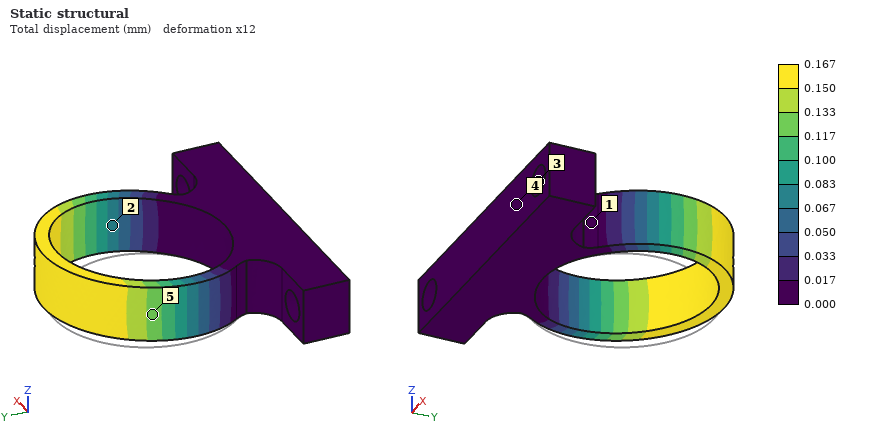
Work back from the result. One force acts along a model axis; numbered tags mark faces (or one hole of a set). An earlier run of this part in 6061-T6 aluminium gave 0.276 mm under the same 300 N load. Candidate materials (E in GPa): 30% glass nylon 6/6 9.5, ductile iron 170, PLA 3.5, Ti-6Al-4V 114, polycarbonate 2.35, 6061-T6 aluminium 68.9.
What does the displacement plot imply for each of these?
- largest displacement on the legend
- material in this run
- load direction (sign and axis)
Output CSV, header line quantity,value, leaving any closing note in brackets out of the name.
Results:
quantity,value
largest displacement on the legend,0.167 mm
material in this run,Ti-6Al-4V
load direction,+X
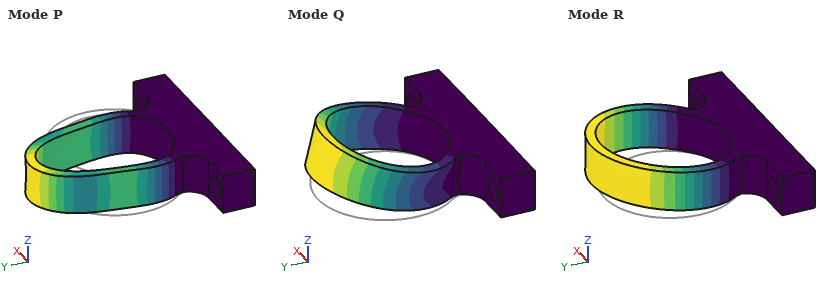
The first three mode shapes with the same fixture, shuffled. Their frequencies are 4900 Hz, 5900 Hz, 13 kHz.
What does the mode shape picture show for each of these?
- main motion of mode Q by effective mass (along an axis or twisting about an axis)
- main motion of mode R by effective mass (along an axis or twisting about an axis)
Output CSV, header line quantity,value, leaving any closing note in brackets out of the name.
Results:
quantity,value
main motion of mode Q by effective mass,along Z
main motion of mode R by effective mass,along X
